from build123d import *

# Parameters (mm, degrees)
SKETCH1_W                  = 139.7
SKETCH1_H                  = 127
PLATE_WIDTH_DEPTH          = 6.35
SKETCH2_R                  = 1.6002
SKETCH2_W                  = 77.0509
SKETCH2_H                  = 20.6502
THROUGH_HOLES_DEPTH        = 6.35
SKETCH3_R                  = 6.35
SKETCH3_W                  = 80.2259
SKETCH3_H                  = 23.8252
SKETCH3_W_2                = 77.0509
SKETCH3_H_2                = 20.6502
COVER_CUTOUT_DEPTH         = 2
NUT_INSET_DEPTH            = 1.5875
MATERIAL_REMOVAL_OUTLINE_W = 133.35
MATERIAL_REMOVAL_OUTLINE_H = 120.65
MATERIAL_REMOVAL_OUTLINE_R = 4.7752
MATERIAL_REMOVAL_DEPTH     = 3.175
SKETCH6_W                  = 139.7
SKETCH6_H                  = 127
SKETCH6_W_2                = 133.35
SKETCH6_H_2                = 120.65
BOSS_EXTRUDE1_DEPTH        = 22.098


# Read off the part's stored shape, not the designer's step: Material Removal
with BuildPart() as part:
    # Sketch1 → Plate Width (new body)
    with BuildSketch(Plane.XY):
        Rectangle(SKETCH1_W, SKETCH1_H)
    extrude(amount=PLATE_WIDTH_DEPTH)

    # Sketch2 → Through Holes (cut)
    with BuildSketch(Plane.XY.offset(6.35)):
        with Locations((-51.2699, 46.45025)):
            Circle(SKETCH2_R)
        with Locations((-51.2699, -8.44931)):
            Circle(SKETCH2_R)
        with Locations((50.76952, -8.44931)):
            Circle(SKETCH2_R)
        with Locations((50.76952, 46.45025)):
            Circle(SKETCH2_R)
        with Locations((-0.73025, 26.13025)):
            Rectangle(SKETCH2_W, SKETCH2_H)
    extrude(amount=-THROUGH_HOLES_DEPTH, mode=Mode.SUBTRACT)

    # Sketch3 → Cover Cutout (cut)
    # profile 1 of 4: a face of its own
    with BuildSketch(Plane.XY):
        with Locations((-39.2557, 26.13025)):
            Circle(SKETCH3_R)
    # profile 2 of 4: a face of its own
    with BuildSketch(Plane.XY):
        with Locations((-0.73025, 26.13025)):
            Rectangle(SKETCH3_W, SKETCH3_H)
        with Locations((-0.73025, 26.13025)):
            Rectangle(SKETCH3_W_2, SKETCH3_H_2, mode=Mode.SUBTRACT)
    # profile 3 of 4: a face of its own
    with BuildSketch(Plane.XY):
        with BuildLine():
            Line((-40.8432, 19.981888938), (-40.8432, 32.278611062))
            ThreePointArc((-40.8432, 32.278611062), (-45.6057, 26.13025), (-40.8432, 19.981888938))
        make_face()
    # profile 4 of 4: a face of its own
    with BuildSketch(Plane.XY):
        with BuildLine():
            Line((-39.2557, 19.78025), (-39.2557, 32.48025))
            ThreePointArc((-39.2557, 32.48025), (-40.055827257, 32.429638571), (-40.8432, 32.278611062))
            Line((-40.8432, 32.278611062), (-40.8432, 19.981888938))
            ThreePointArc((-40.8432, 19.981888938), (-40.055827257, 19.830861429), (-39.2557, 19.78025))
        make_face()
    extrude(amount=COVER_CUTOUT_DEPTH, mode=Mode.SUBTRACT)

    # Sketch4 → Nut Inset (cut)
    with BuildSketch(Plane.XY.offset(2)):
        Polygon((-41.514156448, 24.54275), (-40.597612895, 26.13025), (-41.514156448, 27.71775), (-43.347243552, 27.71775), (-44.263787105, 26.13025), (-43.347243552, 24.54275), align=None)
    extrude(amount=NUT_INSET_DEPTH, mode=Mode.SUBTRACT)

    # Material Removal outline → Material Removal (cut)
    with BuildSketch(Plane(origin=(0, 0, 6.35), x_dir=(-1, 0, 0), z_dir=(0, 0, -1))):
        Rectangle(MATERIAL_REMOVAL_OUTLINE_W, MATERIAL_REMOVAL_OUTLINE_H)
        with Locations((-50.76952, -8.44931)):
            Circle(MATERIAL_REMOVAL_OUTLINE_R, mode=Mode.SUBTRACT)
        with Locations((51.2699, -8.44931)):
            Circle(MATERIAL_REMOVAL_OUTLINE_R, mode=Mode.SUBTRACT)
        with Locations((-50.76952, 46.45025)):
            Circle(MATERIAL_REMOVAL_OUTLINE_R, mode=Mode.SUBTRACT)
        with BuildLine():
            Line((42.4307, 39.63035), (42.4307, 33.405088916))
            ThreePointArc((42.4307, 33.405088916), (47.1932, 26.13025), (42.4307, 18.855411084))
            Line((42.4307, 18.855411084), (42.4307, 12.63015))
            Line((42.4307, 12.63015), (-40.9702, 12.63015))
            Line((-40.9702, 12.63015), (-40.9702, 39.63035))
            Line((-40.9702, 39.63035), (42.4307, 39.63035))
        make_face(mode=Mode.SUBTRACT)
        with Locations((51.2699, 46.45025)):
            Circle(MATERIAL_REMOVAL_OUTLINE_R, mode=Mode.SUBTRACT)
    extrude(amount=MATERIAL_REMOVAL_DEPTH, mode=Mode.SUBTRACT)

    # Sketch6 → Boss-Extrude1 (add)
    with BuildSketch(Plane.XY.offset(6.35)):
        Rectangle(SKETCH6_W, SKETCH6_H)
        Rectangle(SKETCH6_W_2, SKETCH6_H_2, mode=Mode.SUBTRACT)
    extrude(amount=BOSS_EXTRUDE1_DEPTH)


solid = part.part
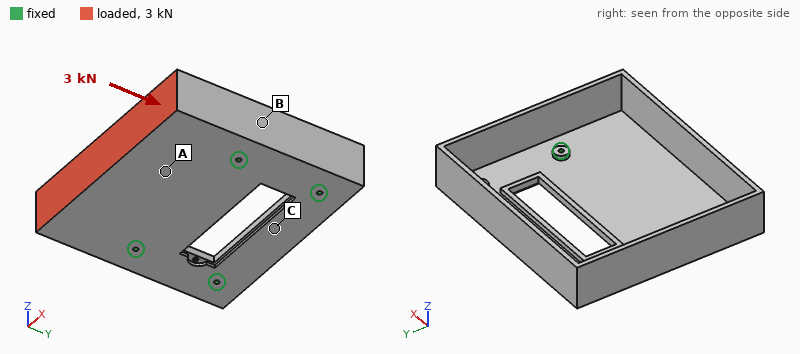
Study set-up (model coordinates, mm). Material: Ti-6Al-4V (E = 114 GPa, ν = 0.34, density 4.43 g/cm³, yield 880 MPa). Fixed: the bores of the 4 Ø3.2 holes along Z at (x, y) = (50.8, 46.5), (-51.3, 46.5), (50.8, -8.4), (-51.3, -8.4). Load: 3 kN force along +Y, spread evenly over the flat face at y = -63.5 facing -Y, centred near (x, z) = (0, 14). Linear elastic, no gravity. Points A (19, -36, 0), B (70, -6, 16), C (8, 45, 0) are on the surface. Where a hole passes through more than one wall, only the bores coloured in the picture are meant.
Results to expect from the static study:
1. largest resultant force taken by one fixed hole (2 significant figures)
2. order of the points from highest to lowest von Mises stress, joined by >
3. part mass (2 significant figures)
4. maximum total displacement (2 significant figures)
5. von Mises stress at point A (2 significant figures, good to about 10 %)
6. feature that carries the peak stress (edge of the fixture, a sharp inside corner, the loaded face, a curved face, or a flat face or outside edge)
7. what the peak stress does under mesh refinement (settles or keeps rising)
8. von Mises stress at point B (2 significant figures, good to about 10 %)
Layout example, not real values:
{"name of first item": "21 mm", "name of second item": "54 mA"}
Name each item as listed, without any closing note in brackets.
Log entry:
{"largest resultant force taken by one fixed hole": "1.1 kN", "order of the points from highest to lowest von Mises stress, joined by >": "A > B > C", "part mass": "420 g", "maximum total displacement": "0.42 mm", "von Mises stress at point A": "34 MPa", "feature that carries the peak stress": "edge of the fixture", "what the peak stress does under mesh refinement": "keeps rising", "von Mises stress at point B": "19 MPa"}
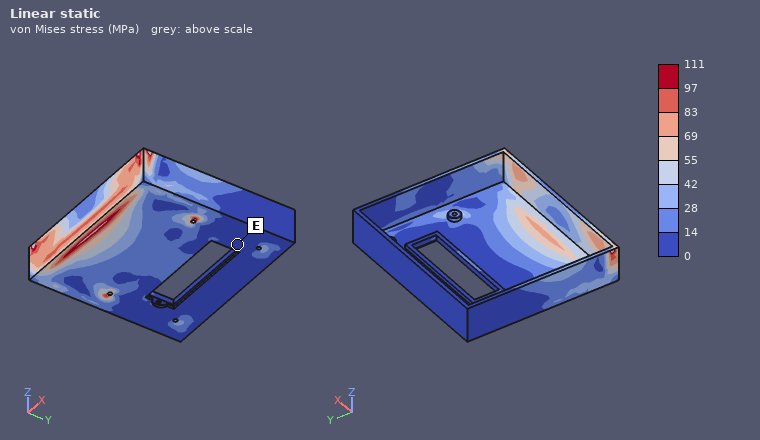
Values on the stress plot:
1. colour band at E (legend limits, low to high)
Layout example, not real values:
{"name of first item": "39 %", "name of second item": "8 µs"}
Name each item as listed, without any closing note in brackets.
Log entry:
{"colour band at E": "0 to 14 MPa"}
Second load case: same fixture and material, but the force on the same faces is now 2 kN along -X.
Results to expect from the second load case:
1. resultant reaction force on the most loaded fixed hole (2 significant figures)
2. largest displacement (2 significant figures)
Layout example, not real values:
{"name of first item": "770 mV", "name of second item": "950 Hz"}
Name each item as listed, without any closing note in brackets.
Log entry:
{"resultant reaction force on the most loaded fixed hole": "1.4 kN", "largest displacement": "98 µm"}
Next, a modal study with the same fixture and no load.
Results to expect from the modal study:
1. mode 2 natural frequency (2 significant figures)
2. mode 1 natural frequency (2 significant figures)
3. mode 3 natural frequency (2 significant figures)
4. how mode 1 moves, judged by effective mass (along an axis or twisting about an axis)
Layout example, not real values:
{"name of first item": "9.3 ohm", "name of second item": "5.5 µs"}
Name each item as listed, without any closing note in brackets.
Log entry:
{"mode 2 natural frequency": "1400 Hz", "mode 1 natural frequency": "1100 Hz", "mode 3 natural frequency": "1900 Hz", "how mode 1 moves, judged by effective mass": "along Z"}
